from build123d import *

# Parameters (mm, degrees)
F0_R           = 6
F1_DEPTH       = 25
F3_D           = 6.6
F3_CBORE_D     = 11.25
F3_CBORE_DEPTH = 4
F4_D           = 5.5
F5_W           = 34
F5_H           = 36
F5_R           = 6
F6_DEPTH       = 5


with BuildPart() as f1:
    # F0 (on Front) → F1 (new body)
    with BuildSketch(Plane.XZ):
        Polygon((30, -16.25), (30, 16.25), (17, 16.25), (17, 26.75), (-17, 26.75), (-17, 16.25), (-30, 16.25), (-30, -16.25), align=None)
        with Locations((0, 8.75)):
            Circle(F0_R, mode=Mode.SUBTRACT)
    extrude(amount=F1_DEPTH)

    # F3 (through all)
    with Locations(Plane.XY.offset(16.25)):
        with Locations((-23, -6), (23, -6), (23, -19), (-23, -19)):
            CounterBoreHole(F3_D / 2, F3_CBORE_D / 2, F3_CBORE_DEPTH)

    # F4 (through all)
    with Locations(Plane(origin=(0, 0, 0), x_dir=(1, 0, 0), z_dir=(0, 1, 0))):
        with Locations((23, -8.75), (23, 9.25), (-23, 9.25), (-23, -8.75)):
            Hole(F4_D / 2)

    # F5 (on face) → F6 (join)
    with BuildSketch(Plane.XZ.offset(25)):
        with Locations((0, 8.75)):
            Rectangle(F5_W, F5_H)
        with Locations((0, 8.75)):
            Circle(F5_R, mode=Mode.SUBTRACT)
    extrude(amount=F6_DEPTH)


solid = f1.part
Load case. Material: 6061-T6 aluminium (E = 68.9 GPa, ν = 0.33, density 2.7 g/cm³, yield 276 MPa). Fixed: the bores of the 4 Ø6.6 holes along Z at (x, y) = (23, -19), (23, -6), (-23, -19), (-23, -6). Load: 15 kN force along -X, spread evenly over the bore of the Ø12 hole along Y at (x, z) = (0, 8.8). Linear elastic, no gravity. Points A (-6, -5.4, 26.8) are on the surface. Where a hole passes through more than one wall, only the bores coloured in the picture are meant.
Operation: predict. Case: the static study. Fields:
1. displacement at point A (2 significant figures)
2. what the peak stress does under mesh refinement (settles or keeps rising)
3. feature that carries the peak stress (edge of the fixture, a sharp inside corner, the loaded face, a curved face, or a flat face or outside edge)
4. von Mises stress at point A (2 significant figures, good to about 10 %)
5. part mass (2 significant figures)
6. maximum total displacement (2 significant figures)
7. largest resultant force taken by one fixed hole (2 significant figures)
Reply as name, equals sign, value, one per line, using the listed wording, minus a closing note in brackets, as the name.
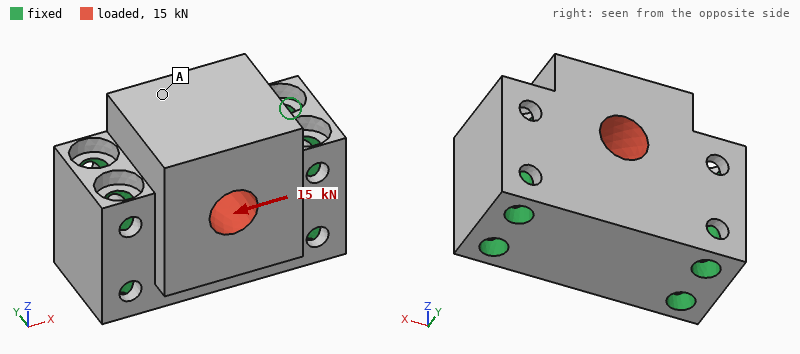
displacement at point A = 4.0 µm
what the peak stress does under mesh refinement = keeps rising
feature that carries the peak stress = edge of the fixture
von Mises stress at point A = 4.5 MPa
part mass = 140 g
maximum total displacement = 6.6 µm
largest resultant force taken by one fixed hole = 4.3 kN
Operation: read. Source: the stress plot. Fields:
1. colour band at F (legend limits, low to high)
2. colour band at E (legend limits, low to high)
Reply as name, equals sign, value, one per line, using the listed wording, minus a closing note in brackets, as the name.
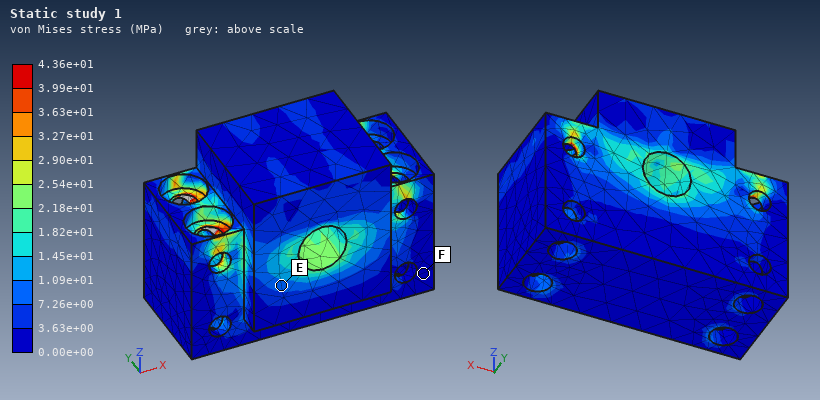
colour band at F = 0.00e+00 to 3.63e+00 MPa
colour band at E = 7.26e+00 to 1.09e+01 MPa
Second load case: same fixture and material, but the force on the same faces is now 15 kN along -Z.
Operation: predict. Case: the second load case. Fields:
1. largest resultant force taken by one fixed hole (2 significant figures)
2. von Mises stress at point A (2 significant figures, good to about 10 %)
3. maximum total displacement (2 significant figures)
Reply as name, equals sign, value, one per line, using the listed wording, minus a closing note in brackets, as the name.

largest resultant force taken by one fixed hole = 4.5 kN
von Mises stress at point A = 10 MPa
maximum total displacement = 10 µm
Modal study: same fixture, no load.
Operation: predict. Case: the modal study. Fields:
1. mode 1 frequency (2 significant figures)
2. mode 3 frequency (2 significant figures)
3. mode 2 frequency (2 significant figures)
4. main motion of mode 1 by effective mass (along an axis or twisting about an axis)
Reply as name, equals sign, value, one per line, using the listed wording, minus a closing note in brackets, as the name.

mode 1 frequency = 17 kHz
mode 3 frequency = 29 kHz
mode 2 frequency = 28 kHz
main motion of mode 1 by effective mass = along Y
